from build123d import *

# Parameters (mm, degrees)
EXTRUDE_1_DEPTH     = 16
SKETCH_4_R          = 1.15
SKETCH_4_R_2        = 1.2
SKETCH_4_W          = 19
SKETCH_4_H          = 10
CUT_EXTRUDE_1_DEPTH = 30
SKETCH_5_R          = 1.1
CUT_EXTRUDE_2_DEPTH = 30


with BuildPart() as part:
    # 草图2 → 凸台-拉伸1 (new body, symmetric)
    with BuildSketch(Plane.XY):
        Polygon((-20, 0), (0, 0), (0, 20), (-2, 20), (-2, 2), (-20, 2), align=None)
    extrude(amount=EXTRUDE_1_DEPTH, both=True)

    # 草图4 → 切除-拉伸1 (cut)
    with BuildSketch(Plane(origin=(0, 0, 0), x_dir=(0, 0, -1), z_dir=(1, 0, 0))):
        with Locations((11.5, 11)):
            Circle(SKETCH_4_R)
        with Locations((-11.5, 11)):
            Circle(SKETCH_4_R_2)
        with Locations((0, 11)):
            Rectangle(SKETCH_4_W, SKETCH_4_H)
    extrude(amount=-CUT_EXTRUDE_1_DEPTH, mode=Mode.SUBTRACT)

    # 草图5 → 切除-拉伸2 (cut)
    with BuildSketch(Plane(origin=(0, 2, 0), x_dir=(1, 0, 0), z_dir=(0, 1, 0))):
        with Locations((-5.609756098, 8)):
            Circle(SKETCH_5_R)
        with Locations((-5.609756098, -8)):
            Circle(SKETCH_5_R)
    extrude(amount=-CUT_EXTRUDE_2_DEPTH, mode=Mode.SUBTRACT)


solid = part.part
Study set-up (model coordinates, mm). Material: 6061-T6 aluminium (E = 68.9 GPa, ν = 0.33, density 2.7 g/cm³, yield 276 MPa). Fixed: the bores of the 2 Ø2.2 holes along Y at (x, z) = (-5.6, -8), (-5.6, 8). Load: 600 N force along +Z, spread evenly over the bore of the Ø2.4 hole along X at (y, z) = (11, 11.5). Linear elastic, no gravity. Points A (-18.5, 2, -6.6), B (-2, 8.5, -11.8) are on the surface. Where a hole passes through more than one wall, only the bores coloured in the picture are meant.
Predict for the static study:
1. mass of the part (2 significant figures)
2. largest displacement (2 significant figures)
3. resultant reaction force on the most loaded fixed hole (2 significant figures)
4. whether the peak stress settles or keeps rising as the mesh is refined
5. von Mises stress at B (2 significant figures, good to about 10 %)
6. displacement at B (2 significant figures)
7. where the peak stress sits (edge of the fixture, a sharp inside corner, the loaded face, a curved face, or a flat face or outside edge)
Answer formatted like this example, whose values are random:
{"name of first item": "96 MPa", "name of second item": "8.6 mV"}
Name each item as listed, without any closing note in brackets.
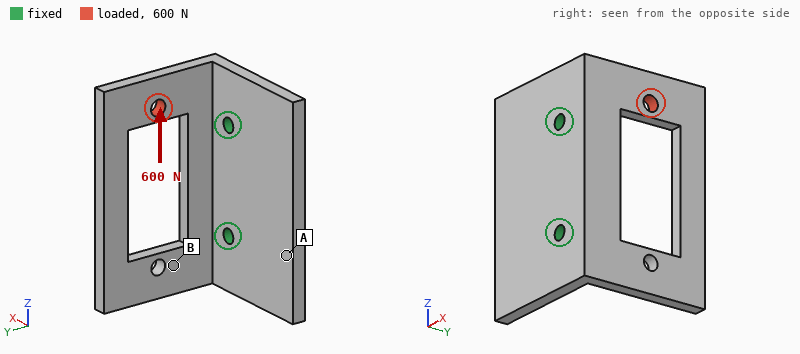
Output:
{"mass of the part": "5.5 g", "largest displacement": "0.14 mm", "resultant reaction force on the most loaded fixed hole": "460 N", "whether the peak stress settles or keeps rising as the mesh is refined": "keeps rising", "von Mises stress at B": "54 MPa", "displacement at B": "0.050 mm", "where the peak stress sits": "edge of the fixture"}
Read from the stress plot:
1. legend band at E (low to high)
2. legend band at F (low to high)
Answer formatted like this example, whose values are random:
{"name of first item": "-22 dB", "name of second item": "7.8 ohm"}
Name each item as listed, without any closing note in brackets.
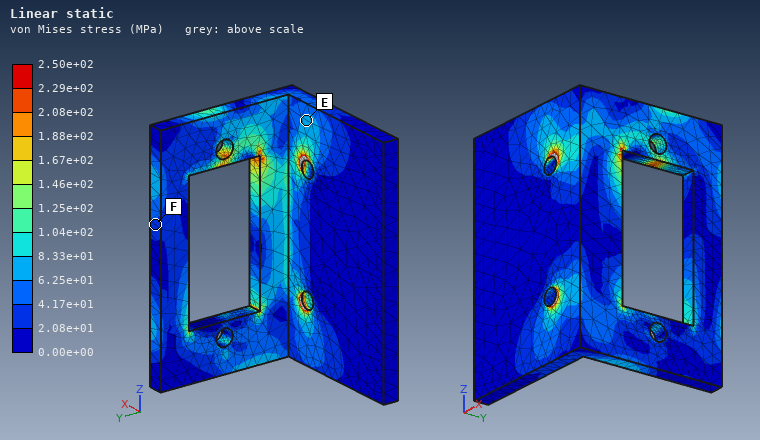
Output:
{"legend band at E": "6.25e+01 to 8.33e+01 MPa", "legend band at F": "2.08e+01 to 4.17e+01 MPa"}
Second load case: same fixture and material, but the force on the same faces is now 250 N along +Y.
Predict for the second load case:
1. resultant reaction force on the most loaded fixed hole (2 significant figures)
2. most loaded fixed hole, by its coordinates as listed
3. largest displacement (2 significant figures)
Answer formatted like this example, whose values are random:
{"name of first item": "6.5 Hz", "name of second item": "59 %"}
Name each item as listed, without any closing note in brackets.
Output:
{"resultant reaction force on the most loaded fixed hole": "280 N", "most loaded fixed hole, by its coordinates as listed": "(-5.6, 8)", "largest displacement": "83 µm"}
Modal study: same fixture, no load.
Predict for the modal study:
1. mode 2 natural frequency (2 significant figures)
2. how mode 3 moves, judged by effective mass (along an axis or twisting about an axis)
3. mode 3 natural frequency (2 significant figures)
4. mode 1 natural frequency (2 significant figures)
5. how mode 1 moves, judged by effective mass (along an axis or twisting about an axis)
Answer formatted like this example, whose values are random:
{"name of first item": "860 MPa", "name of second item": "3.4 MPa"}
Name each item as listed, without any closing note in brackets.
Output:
{"mode 2 natural frequency": "5100 Hz", "how mode 3 moves, judged by effective mass": "along Y", "mode 3 natural frequency": "7300 Hz", "mode 1 natural frequency": "2900 Hz", "how mode 1 moves, judged by effective mass": "along X"}
